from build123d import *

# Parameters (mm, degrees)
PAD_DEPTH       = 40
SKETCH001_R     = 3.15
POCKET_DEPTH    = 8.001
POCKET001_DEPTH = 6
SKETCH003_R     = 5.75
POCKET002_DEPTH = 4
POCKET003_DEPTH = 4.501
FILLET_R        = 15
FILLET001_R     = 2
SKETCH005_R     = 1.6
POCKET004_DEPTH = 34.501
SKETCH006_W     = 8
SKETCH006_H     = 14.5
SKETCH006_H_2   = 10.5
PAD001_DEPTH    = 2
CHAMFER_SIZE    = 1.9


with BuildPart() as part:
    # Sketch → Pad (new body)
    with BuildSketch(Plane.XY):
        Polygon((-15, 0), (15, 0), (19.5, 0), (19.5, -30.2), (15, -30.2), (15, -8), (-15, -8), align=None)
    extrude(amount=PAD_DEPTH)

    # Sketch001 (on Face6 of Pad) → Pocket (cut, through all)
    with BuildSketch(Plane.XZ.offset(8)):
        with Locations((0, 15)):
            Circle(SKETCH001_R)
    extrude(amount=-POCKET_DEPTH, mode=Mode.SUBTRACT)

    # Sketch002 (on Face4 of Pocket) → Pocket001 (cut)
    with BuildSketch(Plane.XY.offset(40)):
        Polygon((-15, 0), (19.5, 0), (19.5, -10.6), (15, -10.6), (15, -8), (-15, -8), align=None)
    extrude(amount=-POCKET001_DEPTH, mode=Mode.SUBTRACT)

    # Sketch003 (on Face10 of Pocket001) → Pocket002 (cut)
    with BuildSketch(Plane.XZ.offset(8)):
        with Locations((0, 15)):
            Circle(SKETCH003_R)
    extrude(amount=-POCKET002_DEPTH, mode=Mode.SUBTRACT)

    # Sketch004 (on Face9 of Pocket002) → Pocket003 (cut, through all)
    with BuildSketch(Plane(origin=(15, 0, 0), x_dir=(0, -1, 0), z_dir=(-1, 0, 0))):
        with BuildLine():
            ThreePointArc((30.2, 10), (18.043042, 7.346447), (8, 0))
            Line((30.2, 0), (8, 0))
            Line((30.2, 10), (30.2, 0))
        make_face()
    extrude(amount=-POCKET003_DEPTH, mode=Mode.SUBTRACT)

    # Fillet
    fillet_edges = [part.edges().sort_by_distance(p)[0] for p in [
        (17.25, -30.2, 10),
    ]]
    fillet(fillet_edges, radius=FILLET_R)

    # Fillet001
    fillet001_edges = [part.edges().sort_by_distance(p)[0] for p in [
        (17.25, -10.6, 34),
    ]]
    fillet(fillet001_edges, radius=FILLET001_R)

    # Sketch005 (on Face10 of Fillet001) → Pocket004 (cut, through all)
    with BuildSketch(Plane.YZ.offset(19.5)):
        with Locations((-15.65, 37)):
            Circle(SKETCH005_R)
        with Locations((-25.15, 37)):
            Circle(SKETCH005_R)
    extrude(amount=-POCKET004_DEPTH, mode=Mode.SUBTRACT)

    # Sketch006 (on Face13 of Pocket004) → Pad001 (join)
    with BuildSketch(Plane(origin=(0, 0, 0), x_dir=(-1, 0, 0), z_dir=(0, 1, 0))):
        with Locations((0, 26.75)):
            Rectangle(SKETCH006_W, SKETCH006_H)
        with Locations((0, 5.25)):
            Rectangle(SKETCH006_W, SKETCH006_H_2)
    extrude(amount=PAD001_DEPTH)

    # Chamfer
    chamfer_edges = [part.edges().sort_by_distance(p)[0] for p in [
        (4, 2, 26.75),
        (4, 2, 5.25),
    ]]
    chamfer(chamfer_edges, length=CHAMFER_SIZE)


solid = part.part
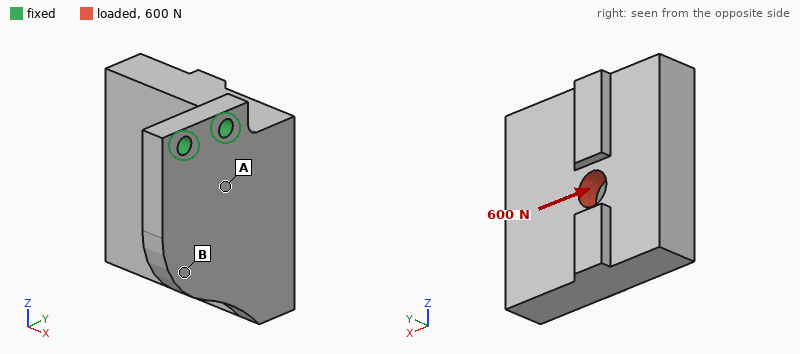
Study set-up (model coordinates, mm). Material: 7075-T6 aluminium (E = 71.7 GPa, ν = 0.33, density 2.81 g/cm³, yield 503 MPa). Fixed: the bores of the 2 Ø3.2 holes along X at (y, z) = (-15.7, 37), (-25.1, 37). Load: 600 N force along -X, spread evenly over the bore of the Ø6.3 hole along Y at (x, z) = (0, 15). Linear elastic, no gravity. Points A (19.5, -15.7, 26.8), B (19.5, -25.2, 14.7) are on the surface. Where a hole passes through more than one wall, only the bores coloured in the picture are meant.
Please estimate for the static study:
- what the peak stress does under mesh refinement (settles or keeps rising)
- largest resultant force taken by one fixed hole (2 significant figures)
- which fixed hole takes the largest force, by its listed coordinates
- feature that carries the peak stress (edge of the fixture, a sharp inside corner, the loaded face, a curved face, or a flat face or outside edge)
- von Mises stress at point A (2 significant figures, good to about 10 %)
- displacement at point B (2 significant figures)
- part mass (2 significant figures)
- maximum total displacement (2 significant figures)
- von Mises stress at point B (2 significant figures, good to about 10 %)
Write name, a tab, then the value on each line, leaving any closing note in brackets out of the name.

what the peak stress does under mesh refinement	keeps rising
largest resultant force taken by one fixed hole	980 N
which fixed hole takes the largest force, by its listed coordinates	(-15.7, 37)
feature that carries the peak stress	edge of the fixture
von Mises stress at point A	120 MPa
displacement at point B	0.12 mm
part mass	34 g
maximum total displacement	0.70 mm
von Mises stress at point B	52 MPa
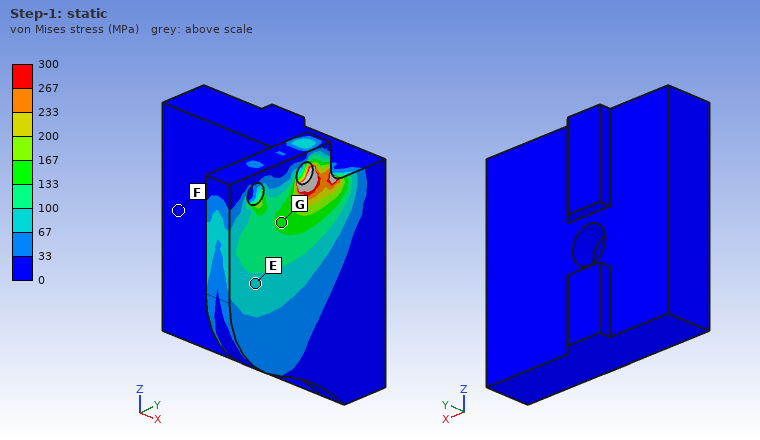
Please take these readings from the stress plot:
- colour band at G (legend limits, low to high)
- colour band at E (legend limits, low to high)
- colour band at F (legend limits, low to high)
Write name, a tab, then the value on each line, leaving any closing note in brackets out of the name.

colour band at G	133 to 167 MPa
colour band at E	67 to 100 MPa
colour band at F	0 to 33 MPa
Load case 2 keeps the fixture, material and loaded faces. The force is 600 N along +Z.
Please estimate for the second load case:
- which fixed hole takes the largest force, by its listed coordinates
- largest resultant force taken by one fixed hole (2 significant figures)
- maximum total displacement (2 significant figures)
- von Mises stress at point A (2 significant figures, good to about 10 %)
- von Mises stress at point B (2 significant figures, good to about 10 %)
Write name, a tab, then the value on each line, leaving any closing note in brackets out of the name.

which fixed hole takes the largest force, by its listed coordinates	(-15.7, 37)
largest resultant force taken by one fixed hole	1.2 kN
maximum total displacement	0.54 mm
von Mises stress at point A	85 MPa
von Mises stress at point B	36 MPa
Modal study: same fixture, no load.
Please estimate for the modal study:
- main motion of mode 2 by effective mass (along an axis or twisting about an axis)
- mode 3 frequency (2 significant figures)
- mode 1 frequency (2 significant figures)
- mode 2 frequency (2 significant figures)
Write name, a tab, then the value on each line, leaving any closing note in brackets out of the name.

main motion of mode 2 by effective mass	along Y
mode 3 frequency	5500 Hz
mode 1 frequency	1000 Hz
mode 2 frequency	1600 Hz
